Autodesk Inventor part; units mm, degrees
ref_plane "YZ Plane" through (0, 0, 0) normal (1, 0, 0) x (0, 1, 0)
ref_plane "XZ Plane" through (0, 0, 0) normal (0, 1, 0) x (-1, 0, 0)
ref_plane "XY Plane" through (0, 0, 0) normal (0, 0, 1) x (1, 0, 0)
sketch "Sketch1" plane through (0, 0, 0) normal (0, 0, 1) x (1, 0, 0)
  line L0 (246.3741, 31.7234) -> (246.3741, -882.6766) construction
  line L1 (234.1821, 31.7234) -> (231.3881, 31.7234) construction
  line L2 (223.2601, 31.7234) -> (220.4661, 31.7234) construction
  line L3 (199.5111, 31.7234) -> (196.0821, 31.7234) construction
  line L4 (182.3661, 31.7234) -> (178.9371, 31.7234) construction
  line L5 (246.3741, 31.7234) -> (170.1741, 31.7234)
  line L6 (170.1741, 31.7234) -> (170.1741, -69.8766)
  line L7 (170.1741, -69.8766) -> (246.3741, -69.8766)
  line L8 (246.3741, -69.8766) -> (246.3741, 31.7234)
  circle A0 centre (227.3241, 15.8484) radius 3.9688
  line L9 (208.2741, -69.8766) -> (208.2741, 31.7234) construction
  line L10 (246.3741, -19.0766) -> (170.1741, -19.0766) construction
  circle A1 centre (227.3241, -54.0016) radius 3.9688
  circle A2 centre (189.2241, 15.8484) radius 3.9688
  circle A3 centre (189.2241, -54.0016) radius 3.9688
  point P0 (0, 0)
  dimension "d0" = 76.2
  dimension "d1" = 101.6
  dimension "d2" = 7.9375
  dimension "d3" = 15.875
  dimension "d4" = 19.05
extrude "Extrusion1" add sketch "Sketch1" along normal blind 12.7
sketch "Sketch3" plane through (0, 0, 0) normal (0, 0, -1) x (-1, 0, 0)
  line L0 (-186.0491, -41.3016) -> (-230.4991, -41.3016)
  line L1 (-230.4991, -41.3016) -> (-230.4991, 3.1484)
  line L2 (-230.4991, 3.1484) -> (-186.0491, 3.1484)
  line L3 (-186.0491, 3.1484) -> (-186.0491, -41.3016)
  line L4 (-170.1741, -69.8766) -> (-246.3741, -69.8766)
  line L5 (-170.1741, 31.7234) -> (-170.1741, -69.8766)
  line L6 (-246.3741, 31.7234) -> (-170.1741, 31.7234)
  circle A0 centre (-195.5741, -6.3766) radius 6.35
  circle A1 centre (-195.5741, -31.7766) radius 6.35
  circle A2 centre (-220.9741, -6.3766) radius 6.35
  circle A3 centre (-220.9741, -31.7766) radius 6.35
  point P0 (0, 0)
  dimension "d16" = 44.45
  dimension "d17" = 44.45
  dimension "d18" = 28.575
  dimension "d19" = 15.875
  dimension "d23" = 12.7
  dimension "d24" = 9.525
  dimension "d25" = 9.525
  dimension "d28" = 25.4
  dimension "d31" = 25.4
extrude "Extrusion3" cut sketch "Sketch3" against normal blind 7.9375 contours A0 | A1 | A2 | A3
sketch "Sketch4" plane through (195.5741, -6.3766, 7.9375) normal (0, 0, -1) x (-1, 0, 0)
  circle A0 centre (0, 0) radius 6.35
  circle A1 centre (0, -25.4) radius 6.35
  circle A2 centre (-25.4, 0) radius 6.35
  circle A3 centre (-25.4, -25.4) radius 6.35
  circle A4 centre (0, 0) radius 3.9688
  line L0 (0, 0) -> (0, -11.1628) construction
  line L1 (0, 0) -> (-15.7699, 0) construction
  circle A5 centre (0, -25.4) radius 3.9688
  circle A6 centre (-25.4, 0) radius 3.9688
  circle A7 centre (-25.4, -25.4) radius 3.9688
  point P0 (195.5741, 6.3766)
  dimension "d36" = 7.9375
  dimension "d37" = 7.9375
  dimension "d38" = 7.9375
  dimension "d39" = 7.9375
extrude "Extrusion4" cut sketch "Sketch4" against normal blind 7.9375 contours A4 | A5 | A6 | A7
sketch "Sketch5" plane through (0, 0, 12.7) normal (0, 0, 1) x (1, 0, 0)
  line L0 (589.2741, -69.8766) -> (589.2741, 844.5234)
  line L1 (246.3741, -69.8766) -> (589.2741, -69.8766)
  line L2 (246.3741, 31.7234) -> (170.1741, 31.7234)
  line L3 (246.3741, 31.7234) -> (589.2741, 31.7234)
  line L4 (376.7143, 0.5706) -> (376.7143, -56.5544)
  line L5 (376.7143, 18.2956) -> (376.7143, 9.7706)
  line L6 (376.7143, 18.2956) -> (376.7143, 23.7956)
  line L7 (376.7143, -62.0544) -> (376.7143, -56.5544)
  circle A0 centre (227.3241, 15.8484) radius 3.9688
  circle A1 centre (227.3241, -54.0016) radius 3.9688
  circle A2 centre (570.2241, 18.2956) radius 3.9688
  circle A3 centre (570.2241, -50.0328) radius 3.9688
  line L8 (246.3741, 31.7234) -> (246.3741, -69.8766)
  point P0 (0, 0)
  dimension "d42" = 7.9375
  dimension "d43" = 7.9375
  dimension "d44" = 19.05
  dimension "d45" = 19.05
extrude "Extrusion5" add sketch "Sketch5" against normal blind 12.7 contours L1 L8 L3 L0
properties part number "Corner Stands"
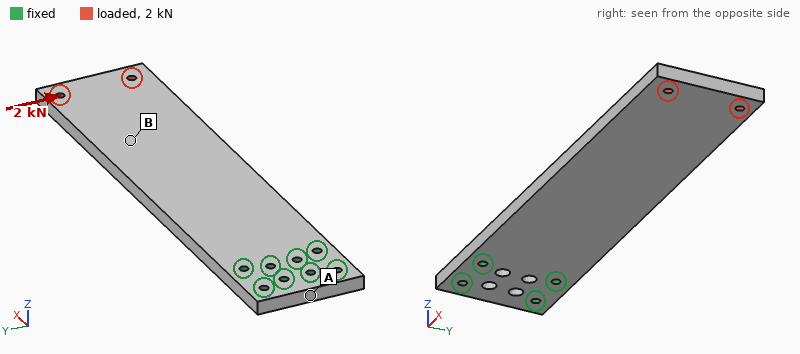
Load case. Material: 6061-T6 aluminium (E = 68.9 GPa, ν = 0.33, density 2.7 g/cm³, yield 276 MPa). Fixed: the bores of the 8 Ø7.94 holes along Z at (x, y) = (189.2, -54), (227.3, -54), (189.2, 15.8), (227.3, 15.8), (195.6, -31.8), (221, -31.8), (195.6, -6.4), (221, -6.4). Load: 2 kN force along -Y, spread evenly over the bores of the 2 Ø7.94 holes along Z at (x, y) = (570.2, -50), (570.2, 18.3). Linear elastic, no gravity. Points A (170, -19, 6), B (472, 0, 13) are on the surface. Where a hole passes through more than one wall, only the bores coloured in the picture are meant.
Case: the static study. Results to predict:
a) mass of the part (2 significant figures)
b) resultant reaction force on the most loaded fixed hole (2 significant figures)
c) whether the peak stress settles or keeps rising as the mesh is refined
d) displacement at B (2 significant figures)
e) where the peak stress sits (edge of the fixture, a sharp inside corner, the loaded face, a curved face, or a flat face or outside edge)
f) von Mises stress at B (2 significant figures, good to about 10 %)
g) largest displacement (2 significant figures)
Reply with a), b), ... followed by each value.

a) 1.4 kg
b) 7.8 kN
c) keeps rising
d) 0.23 mm
e) edge of the fixture
f) 4.9 MPa
g) 0.43 mm
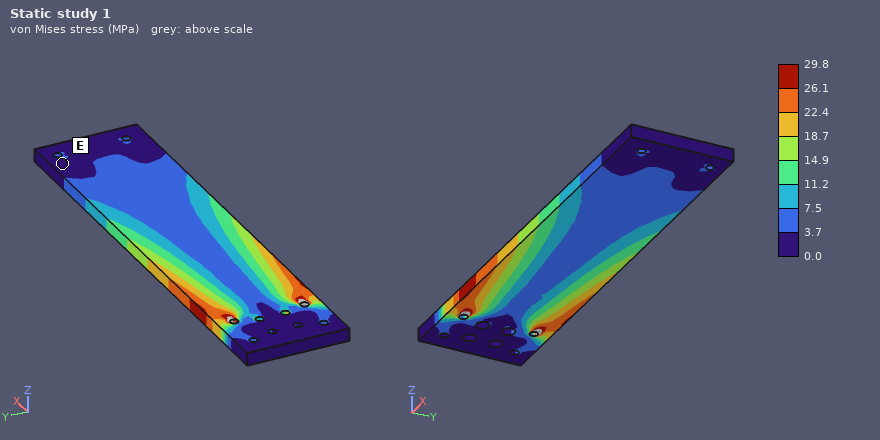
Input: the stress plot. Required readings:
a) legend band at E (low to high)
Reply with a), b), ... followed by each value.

a) 0.0 to 3.7 MPa
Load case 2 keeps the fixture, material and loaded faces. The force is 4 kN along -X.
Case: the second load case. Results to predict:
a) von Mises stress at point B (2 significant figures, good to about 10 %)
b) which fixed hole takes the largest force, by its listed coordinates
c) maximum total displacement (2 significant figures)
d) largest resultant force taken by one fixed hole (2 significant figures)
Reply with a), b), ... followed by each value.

a) 3.3 MPa
b) (227.3, 15.8)
c) 25 µm
d) 1.4 kN
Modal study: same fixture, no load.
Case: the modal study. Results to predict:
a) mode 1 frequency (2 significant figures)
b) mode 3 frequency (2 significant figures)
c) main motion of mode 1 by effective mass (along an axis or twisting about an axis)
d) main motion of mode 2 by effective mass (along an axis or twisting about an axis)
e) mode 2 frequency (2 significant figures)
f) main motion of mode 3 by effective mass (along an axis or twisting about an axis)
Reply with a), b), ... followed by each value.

a) 79 Hz
b) 550 Hz
c) along Z
d) along Z
e) 490 Hz
f) twisting about X
